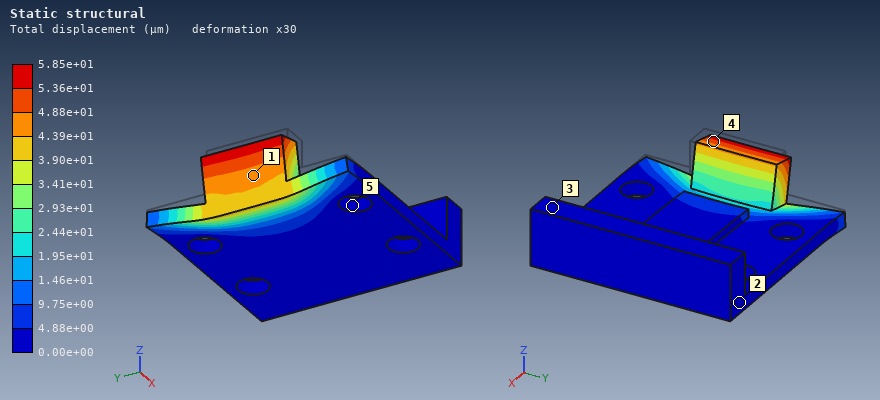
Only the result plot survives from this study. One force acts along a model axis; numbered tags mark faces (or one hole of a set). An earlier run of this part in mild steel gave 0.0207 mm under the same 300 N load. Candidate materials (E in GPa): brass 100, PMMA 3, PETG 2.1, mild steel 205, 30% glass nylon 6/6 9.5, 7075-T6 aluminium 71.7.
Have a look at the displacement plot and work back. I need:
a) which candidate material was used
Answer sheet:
7075-T6 aluminium
